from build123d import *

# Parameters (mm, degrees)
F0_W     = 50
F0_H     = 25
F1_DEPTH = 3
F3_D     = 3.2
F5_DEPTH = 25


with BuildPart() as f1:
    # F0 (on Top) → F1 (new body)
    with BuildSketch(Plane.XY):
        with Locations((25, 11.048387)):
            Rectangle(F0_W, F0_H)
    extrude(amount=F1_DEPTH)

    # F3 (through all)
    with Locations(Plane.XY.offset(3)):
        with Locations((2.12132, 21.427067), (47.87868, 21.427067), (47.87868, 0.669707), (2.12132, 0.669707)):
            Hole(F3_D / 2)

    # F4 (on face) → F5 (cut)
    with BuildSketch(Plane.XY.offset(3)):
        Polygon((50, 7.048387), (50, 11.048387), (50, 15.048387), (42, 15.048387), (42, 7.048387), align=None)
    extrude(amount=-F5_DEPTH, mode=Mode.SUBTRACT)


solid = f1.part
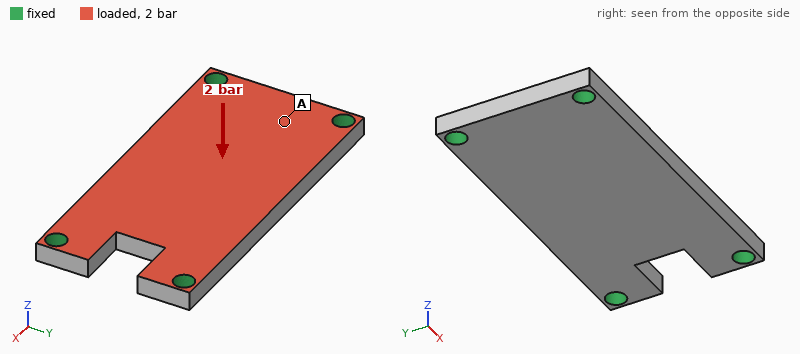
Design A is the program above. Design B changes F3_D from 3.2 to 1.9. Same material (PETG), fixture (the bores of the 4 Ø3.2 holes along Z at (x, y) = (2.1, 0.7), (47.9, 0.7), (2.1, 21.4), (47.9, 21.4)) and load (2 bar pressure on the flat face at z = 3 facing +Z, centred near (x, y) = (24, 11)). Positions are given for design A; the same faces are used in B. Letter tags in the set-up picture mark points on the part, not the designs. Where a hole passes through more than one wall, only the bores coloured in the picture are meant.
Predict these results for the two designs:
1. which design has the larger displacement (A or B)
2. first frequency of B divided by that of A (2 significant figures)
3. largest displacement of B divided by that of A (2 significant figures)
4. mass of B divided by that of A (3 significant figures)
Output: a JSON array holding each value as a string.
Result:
["B", "0.91", "1.2", "1.02"]
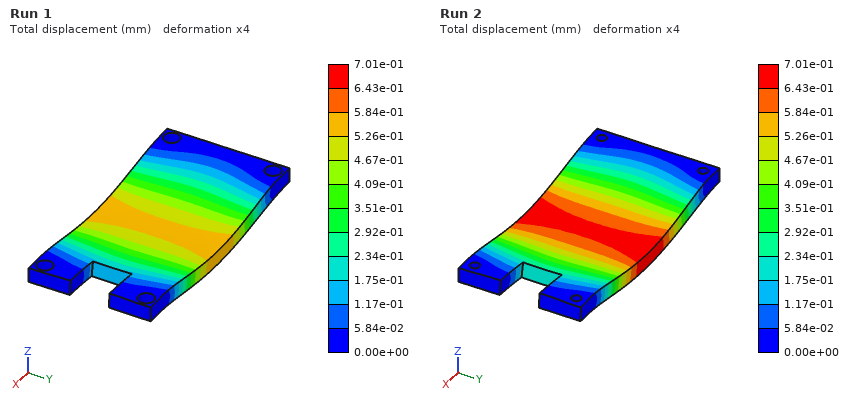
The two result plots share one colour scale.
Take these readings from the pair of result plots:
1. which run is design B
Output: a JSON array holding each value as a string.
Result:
["Run 2"]
